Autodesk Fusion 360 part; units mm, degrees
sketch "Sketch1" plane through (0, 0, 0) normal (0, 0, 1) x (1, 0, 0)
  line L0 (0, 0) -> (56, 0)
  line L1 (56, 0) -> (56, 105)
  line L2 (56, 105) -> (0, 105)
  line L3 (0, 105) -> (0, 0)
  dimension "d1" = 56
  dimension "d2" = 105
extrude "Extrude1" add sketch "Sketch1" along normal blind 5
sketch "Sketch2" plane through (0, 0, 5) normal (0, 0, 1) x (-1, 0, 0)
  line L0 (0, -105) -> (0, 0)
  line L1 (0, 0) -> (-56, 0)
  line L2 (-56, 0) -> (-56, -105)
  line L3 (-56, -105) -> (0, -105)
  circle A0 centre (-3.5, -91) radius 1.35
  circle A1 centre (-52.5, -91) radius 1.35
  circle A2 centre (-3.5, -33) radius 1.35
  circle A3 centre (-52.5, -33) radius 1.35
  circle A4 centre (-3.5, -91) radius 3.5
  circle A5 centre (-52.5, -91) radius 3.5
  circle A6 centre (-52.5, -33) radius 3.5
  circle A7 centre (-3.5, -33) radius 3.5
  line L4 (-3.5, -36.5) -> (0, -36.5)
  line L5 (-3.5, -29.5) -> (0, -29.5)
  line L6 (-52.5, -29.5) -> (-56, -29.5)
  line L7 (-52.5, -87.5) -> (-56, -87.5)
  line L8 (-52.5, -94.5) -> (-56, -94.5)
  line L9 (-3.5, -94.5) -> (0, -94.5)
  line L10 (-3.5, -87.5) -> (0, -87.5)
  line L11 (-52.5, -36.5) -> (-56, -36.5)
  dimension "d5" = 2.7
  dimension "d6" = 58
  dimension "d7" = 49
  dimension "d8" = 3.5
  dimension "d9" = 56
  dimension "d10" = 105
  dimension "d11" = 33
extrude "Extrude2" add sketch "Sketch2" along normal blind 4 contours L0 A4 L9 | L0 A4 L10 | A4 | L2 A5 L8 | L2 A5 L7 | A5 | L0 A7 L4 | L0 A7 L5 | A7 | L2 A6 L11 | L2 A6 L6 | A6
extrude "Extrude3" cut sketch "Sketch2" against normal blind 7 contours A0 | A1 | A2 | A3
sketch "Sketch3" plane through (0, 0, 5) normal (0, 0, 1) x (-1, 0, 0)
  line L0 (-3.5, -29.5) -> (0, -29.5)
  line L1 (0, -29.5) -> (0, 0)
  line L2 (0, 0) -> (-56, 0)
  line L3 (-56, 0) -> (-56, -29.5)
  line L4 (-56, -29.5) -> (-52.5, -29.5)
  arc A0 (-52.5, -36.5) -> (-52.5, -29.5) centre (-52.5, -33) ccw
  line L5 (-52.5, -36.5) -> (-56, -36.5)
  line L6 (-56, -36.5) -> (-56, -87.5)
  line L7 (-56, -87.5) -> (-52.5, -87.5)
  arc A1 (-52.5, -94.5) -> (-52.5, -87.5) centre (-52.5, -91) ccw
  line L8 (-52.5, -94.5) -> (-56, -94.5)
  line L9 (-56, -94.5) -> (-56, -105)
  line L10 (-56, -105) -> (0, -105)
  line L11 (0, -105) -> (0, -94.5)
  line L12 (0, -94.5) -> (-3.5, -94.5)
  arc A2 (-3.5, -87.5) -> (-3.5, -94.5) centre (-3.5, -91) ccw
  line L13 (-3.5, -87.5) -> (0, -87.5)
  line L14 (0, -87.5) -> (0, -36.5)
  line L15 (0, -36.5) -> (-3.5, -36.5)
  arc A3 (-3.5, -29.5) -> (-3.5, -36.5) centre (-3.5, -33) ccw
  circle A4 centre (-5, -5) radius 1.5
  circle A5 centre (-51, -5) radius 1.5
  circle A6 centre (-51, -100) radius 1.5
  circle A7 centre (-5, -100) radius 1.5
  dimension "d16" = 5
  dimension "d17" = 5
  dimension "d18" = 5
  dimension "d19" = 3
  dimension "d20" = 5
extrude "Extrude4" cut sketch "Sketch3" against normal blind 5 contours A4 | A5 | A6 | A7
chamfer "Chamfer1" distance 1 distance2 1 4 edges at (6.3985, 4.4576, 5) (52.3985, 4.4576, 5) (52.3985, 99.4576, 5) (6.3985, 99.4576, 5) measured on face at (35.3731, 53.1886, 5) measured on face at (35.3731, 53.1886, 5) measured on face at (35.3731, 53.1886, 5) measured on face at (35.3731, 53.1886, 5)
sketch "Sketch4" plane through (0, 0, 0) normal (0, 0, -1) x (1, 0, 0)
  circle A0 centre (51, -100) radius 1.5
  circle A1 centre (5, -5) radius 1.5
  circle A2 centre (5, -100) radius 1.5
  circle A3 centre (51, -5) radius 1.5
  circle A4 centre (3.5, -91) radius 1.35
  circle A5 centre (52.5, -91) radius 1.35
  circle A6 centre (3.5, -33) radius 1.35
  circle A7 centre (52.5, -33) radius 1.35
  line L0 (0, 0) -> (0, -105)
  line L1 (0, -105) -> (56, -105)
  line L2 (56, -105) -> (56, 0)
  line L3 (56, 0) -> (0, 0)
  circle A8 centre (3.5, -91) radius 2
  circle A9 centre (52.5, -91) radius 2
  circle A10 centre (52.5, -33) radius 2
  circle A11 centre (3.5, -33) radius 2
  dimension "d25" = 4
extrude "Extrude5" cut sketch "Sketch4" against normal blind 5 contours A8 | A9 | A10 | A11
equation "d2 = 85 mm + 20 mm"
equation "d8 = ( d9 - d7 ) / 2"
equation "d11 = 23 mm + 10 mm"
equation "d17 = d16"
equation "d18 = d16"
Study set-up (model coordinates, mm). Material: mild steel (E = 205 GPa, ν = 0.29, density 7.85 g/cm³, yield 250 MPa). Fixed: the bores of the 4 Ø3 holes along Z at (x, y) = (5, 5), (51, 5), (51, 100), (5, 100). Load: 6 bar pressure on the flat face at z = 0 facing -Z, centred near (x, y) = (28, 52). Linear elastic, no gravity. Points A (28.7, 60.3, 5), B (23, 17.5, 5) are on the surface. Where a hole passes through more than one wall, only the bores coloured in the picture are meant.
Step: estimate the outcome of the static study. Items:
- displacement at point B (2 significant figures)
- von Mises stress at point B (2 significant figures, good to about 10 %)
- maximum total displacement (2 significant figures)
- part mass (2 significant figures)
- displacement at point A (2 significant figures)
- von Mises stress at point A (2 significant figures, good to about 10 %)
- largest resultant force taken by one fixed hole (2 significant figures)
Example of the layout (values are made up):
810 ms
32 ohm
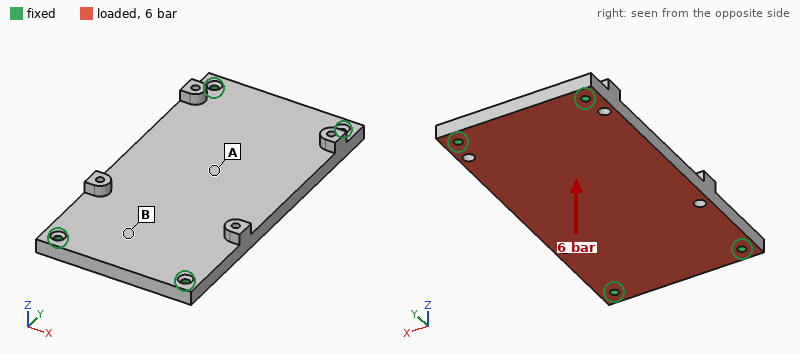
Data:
36 µm
25 MPa
96 µm
230 g
91 µm
58 MPa
890 N
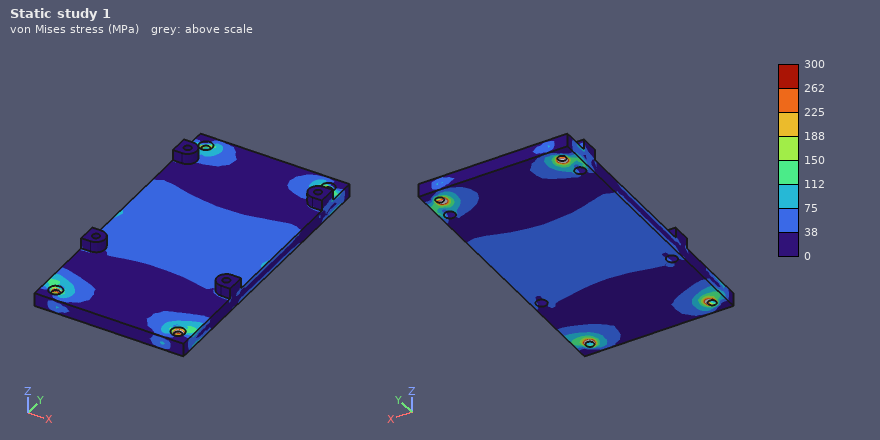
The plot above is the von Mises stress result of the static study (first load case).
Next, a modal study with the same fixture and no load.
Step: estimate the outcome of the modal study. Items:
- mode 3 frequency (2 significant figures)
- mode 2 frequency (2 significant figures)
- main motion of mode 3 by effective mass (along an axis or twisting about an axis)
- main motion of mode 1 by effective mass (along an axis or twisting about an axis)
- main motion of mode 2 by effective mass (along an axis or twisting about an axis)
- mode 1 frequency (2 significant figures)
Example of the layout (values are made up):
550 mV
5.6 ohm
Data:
6200 Hz
4000 Hz
twisting about X
along Z
twisting about Y
2300 Hz
